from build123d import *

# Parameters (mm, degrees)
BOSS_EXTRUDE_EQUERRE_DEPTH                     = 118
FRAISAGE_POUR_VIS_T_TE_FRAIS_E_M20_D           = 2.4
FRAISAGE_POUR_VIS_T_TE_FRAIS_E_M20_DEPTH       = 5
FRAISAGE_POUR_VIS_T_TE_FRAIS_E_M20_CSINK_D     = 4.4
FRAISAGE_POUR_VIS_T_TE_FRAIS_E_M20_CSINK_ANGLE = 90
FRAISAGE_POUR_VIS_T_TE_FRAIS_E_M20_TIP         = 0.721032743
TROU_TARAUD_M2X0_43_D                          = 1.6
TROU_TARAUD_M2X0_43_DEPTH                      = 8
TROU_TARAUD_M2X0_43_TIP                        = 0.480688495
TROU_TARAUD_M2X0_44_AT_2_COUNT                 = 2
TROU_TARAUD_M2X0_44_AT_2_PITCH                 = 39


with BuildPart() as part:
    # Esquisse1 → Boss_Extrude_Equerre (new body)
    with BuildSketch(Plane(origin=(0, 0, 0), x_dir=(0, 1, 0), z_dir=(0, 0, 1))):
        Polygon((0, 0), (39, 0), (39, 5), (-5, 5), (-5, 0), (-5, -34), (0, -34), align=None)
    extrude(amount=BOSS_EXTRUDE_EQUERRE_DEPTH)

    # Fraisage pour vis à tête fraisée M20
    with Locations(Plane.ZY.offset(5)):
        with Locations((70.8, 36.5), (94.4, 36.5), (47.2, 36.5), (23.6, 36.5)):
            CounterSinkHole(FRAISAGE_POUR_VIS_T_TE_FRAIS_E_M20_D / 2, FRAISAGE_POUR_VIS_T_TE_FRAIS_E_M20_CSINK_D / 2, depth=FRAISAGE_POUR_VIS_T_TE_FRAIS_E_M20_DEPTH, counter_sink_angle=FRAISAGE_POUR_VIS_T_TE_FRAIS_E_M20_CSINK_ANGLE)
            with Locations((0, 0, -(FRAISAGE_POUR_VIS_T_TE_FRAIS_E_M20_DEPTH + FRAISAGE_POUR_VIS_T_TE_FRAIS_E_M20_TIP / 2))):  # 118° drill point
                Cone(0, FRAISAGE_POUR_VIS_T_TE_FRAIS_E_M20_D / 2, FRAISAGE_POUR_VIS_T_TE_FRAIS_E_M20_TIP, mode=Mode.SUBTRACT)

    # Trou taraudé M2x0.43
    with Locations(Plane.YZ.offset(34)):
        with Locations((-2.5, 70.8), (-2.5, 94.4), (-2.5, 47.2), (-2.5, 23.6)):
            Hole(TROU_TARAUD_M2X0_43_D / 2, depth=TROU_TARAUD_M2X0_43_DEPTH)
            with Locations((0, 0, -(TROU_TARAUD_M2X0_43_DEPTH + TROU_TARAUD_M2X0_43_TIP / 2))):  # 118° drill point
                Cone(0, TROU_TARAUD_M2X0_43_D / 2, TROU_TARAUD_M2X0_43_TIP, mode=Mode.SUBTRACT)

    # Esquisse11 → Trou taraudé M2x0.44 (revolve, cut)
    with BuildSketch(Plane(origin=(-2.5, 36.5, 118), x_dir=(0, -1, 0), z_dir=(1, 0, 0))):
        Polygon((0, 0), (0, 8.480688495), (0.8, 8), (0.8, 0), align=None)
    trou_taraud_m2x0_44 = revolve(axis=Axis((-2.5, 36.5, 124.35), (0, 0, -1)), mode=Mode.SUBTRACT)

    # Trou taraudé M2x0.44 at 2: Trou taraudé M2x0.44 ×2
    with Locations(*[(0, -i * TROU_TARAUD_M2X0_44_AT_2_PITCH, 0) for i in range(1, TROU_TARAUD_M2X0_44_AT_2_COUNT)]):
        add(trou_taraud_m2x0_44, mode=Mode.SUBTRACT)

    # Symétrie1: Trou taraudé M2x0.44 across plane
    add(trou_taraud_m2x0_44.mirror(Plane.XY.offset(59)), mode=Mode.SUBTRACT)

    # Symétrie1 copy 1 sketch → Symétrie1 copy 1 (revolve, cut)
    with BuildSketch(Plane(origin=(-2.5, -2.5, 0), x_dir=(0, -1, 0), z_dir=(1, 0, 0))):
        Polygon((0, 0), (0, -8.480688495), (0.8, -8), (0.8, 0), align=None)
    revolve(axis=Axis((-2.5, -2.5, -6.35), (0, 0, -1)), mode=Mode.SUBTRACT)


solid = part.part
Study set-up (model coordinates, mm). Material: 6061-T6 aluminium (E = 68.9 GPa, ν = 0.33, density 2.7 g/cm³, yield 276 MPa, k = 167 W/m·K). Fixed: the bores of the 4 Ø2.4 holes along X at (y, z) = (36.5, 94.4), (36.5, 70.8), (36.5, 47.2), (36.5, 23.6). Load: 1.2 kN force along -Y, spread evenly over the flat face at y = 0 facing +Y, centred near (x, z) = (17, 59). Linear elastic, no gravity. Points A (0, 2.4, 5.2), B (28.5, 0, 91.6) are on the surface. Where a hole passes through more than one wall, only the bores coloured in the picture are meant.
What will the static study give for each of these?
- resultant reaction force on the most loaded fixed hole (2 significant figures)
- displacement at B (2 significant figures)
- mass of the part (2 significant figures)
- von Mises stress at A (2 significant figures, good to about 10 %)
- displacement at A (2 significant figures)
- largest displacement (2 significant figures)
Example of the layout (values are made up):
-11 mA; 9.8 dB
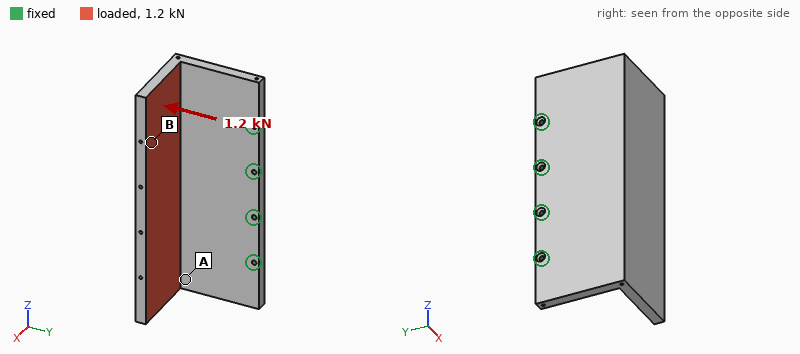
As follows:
340 N; 0.54 mm; 120 g; 38 MPa; 0.25 mm; 0.65 mm
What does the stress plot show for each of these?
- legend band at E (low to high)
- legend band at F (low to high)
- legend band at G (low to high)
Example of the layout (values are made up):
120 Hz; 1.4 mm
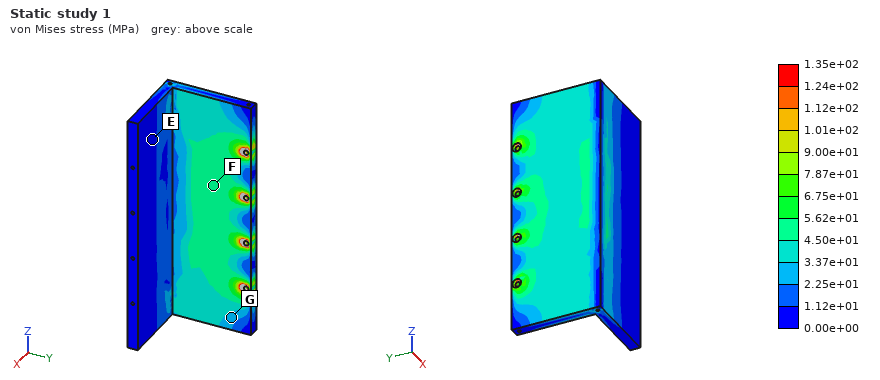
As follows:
0.00e+00 to 1.12e+01 MPa; 4.50e+01 to 5.62e+01 MPa; 2.25e+01 to 3.37e+01 MPa
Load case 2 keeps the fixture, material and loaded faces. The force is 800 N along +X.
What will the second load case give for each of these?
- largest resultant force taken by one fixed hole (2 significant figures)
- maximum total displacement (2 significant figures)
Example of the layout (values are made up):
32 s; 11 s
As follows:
210 N; 0.47 mm
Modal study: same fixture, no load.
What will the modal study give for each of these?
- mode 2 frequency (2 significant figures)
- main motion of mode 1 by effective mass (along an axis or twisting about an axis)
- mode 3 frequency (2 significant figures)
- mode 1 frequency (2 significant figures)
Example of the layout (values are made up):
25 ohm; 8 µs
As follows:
1200 Hz; along X; 2500 Hz; 760 Hz
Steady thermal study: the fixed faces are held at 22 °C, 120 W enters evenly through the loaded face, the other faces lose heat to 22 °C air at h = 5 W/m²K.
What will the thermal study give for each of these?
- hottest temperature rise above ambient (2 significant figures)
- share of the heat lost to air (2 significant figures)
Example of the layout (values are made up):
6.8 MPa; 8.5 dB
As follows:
79 K; 3.2 %
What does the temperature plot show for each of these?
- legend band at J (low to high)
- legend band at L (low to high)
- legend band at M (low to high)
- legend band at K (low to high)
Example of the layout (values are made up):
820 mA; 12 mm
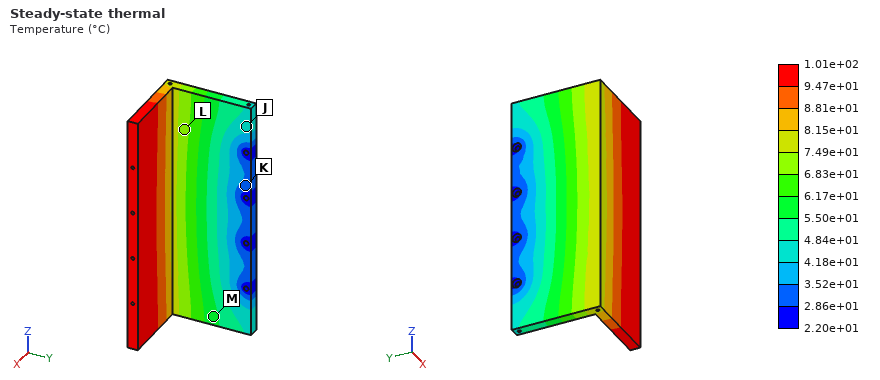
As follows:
4.18e+01 to 4.84e+01 °C; 6.83e+01 to 7.49e+01 °C; 5.50e+01 to 6.17e+01 °C; 2.86e+01 to 3.52e+01 °C
